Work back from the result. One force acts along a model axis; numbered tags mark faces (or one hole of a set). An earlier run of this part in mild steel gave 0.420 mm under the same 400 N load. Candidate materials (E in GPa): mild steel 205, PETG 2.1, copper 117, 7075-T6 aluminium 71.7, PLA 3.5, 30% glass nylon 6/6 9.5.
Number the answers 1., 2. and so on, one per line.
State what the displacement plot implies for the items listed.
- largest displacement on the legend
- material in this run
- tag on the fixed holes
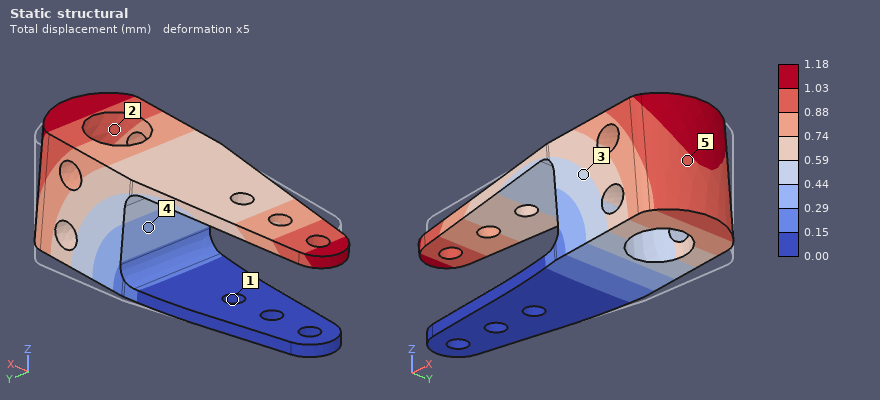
1. 1.18 mm
2. 7075-T6 aluminium
3. 1
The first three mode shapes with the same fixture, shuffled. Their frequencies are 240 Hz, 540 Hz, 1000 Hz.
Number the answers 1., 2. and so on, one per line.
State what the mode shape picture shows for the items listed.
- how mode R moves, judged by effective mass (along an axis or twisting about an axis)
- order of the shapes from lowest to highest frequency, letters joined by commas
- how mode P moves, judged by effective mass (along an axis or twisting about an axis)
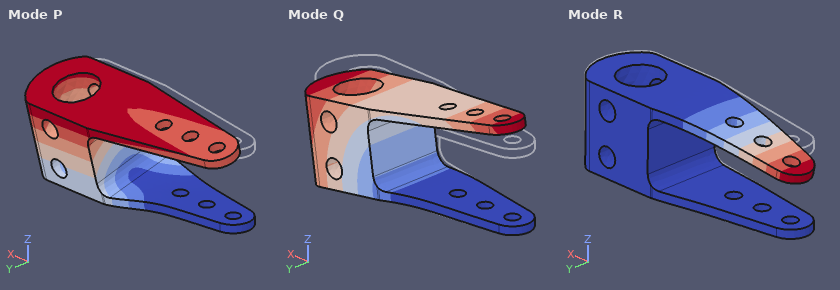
1. along Z
2. Q, P, R
3. along Y
